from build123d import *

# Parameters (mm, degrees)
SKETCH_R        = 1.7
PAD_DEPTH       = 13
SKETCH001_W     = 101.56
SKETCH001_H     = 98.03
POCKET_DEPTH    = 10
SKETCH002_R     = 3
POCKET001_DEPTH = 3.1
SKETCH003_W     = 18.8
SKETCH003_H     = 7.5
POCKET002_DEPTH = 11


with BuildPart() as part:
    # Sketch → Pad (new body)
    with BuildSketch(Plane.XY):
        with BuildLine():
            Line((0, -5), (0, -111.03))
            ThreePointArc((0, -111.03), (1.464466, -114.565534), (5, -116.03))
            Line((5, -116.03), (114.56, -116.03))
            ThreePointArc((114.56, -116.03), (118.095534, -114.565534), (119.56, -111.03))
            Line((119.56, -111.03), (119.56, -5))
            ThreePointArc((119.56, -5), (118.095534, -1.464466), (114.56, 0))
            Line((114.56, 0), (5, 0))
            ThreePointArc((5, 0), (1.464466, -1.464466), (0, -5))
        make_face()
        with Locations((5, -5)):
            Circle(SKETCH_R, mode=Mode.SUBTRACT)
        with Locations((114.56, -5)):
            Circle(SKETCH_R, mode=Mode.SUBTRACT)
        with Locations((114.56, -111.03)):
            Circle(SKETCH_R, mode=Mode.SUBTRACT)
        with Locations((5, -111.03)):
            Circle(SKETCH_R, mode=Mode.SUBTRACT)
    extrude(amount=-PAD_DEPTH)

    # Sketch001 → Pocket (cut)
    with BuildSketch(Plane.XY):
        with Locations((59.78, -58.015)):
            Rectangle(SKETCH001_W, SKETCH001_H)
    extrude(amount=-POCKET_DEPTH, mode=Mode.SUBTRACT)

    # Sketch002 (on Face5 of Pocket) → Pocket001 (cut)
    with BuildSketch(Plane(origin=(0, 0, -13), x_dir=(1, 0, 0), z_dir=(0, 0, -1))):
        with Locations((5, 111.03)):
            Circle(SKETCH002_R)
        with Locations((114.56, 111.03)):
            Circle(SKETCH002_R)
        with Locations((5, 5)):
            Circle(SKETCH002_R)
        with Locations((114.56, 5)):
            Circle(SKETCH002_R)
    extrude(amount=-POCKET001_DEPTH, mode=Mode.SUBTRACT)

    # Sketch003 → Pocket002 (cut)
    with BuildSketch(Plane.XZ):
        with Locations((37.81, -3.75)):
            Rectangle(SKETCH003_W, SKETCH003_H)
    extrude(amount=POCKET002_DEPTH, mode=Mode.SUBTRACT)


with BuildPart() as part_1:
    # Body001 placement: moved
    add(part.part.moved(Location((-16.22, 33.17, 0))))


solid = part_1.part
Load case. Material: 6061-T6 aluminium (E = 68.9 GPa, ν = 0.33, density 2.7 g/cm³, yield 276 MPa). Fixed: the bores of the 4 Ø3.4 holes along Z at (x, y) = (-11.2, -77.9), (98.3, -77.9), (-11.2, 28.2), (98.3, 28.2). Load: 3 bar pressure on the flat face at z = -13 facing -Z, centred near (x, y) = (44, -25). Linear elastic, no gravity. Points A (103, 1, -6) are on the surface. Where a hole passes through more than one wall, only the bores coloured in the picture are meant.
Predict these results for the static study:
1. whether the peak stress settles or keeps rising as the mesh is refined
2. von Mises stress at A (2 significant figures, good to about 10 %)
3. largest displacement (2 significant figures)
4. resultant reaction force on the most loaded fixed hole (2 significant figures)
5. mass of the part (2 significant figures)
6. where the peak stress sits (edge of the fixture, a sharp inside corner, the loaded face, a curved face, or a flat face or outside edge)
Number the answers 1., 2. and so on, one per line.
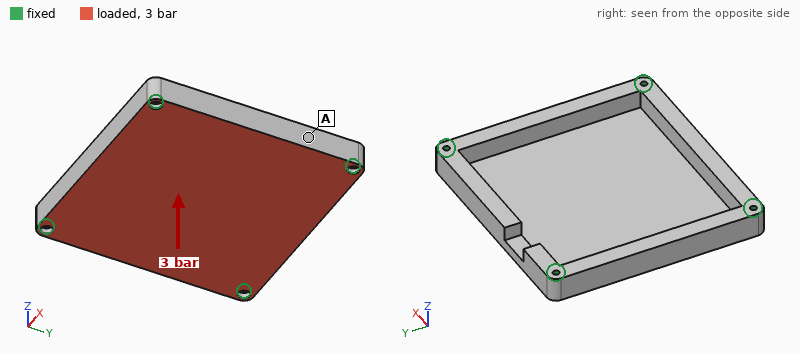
1. keeps rising
2. 16 MPa
3. 0.38 mm
4. 1.8 kN
5. 210 g
6. edge of the fixture
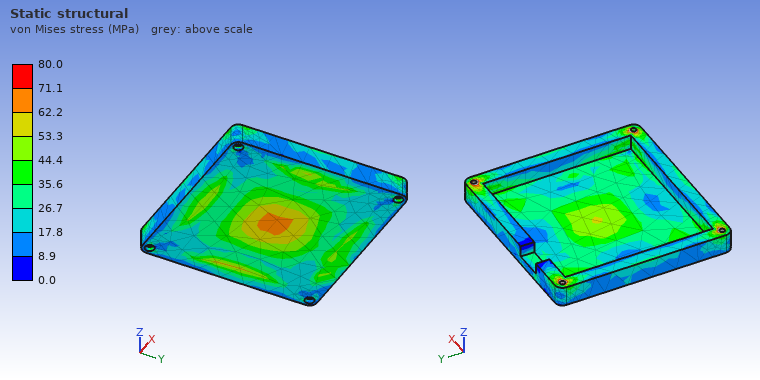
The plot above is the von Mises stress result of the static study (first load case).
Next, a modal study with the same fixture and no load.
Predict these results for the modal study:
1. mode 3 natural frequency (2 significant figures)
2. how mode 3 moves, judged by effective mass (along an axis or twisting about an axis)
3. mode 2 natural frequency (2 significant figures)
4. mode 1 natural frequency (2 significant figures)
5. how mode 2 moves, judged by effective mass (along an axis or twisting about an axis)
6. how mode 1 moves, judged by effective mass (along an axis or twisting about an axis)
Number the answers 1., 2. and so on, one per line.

1. 3700 Hz
2. twisting about Y
3. 3600 Hz
4. 2000 Hz
5. twisting about X
6. along Z
